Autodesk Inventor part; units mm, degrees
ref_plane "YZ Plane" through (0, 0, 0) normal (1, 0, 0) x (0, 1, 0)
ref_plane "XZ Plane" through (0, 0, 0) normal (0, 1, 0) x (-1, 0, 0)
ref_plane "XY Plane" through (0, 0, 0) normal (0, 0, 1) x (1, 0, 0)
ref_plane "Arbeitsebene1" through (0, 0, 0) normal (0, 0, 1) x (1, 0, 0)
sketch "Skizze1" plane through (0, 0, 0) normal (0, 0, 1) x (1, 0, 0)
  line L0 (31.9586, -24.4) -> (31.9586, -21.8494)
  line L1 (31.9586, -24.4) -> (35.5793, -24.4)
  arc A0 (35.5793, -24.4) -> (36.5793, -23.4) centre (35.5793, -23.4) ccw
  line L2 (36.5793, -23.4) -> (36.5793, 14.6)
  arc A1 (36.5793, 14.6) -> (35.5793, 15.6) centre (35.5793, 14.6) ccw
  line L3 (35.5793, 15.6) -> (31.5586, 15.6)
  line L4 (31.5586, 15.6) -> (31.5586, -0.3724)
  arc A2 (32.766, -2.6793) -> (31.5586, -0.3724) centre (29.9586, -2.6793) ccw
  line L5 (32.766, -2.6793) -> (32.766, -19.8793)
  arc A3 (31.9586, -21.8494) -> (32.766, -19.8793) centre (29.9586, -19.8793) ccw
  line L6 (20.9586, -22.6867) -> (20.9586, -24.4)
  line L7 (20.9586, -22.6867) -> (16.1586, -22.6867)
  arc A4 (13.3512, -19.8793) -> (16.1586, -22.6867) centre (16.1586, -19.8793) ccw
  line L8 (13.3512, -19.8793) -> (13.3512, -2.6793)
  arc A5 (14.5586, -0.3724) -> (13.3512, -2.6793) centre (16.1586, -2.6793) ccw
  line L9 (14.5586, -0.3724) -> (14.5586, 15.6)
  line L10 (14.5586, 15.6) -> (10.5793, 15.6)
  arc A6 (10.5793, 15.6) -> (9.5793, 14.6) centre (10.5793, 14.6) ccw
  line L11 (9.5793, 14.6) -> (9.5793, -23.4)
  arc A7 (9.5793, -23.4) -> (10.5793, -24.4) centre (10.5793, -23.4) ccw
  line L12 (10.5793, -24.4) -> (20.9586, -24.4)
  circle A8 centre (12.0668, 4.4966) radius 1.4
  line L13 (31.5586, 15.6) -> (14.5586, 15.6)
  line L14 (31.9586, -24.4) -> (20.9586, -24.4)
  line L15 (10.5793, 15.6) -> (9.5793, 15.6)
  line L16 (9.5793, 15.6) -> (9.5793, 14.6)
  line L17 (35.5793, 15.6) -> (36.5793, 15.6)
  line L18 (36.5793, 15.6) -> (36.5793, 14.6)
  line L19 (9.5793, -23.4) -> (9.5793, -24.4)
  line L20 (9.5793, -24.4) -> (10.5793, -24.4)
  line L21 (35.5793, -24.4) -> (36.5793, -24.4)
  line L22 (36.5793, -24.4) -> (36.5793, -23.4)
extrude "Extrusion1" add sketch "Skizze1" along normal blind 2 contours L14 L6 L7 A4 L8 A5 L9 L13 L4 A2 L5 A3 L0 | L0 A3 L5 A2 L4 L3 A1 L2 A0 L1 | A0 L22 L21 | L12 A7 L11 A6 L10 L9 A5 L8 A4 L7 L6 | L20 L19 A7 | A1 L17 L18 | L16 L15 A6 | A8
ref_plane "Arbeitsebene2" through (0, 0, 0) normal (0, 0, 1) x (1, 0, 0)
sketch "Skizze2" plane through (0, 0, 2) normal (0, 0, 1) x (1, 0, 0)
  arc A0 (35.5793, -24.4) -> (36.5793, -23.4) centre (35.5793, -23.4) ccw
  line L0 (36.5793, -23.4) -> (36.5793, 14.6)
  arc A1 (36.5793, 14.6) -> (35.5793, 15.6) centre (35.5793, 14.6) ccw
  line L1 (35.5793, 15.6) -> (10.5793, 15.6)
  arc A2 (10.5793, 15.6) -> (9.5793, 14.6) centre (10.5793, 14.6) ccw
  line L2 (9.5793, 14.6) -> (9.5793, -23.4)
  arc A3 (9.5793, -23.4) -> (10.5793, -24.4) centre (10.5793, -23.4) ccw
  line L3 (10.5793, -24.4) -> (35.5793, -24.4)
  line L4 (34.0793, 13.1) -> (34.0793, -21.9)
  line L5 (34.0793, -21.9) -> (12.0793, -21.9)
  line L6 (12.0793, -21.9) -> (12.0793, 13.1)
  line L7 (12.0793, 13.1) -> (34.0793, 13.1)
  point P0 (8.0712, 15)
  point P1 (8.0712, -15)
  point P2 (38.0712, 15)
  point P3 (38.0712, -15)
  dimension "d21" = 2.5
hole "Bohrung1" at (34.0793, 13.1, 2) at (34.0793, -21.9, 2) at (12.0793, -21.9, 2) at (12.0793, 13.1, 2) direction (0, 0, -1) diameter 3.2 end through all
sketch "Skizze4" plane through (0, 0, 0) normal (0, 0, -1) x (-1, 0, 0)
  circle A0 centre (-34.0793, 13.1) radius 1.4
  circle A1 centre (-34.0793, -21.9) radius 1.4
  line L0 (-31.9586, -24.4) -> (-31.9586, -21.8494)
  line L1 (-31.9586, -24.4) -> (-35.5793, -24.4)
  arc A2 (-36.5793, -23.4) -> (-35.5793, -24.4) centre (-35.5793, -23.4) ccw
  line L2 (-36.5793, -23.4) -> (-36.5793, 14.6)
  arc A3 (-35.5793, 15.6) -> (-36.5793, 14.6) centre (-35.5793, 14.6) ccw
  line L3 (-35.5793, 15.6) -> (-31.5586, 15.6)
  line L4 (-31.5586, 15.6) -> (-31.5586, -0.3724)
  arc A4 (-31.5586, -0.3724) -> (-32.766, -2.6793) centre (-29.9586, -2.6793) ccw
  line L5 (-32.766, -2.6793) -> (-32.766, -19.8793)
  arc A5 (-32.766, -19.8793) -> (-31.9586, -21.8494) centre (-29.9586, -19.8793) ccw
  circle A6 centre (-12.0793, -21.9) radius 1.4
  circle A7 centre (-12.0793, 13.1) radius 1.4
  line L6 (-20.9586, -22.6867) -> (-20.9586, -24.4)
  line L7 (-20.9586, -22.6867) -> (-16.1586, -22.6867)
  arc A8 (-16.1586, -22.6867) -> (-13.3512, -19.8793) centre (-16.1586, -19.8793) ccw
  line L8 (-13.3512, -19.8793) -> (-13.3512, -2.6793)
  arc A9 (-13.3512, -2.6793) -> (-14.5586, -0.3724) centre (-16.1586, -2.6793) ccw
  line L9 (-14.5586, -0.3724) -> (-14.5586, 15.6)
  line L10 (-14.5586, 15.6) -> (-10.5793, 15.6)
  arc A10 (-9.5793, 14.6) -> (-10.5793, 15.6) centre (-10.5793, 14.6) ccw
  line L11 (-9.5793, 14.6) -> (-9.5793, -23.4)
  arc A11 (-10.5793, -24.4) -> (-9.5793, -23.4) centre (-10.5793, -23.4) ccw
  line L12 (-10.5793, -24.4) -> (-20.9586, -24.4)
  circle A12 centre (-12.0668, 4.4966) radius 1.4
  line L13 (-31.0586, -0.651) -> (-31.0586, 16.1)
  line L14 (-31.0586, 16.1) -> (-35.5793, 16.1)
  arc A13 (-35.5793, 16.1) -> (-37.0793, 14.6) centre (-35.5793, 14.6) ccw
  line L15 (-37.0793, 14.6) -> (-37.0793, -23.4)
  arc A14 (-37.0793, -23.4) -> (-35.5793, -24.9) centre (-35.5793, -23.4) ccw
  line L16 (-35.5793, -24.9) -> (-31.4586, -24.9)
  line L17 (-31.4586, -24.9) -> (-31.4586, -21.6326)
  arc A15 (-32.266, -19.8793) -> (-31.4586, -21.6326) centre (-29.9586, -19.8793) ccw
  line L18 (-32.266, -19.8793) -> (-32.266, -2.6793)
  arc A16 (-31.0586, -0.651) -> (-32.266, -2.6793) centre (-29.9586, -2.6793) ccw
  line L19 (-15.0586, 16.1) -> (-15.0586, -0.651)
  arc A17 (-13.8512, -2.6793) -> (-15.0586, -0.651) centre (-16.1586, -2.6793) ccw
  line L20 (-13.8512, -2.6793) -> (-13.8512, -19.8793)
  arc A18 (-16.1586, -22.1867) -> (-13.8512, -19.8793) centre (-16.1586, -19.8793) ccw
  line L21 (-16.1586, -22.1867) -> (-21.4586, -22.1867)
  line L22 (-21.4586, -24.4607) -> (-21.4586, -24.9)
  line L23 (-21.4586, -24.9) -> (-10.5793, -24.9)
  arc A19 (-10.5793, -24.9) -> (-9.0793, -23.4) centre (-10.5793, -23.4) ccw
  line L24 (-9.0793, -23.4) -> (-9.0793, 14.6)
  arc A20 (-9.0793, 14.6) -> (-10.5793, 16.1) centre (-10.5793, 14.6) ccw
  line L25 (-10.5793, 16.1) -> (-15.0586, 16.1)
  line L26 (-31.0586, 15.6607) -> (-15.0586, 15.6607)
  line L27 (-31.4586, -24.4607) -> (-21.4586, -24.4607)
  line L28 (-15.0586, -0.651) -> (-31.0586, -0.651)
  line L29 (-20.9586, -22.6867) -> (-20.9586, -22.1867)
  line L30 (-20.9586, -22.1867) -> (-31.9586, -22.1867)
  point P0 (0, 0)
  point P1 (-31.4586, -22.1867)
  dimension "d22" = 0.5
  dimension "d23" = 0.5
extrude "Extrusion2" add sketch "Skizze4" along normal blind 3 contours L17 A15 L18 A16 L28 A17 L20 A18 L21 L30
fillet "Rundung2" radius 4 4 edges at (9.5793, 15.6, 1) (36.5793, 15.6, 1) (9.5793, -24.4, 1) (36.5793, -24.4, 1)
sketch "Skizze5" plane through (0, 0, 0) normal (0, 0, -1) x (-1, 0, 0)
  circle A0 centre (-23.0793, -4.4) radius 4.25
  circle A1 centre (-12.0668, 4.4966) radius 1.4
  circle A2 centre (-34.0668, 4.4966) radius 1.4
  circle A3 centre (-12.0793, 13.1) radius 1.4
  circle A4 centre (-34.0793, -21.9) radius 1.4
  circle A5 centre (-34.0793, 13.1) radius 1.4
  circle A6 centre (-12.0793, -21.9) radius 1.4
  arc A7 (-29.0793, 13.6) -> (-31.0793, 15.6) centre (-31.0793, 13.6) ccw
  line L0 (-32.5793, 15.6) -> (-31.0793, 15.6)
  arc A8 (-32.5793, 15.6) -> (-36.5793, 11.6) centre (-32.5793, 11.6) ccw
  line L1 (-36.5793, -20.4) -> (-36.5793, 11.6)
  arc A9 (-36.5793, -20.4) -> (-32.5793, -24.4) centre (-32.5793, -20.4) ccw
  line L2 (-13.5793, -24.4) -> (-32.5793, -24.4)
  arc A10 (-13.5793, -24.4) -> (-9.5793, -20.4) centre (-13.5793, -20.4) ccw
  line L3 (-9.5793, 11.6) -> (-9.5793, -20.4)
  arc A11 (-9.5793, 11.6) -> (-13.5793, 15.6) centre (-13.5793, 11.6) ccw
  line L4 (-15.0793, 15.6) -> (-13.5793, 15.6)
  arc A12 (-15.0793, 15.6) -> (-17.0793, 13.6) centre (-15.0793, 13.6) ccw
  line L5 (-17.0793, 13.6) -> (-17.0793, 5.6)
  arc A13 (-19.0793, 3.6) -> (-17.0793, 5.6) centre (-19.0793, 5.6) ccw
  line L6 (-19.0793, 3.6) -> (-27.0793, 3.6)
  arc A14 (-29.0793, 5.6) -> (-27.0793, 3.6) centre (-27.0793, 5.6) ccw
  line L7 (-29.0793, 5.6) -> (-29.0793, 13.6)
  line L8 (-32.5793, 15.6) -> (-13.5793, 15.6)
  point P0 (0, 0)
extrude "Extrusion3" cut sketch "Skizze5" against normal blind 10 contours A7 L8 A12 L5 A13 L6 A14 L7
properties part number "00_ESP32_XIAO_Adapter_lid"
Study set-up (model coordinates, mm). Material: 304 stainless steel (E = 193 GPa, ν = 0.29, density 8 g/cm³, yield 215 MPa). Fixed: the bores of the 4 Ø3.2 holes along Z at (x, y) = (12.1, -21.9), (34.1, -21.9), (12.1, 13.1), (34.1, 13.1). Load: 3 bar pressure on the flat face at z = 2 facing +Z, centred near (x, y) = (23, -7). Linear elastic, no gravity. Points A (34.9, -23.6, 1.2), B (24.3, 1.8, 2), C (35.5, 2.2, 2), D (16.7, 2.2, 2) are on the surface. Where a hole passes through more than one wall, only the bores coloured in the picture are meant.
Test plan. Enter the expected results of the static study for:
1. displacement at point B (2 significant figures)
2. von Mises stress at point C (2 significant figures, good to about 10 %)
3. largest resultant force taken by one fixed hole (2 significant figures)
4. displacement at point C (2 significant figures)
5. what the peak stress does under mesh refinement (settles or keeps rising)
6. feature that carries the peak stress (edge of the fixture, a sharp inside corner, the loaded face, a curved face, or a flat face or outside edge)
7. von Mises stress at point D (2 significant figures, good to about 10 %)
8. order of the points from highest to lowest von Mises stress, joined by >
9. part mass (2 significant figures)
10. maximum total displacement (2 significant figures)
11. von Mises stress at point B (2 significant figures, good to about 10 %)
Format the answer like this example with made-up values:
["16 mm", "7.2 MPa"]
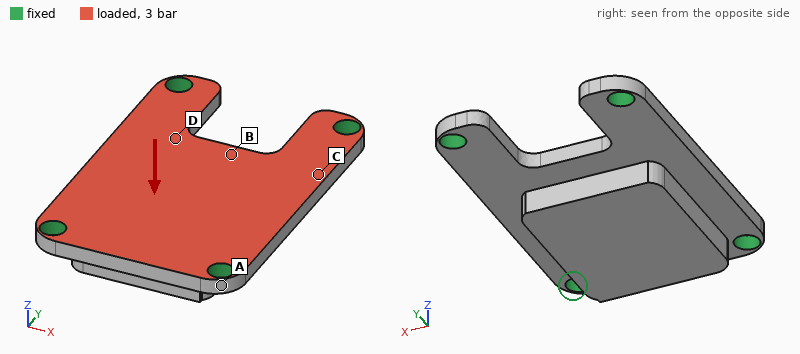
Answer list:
["7.4 µm", "21 MPa", "84 N", "5.6 µm", "keeps rising", "edge of the fixture", "27 MPa", "D > C > B > A", "24 g", "7.6 µm", "12 MPa"]
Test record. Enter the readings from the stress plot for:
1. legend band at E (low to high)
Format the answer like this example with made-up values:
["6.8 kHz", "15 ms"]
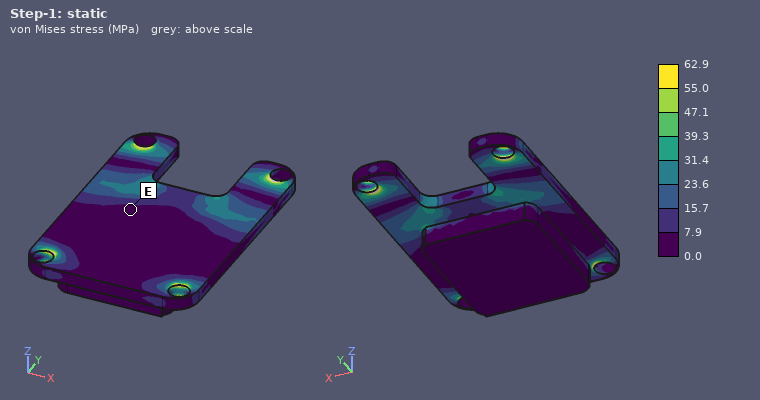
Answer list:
["0.0 to 7.9 MPa"]
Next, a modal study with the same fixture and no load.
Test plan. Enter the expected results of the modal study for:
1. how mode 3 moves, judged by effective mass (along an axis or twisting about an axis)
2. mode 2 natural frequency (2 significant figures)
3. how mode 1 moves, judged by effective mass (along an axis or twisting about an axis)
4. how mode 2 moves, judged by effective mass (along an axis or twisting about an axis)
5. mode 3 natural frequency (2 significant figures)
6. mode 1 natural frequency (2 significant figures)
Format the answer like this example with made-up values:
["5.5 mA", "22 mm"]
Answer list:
["along X", "15 kHz", "along Z", "twisting about Y", "26 kHz", "7300 Hz"]
